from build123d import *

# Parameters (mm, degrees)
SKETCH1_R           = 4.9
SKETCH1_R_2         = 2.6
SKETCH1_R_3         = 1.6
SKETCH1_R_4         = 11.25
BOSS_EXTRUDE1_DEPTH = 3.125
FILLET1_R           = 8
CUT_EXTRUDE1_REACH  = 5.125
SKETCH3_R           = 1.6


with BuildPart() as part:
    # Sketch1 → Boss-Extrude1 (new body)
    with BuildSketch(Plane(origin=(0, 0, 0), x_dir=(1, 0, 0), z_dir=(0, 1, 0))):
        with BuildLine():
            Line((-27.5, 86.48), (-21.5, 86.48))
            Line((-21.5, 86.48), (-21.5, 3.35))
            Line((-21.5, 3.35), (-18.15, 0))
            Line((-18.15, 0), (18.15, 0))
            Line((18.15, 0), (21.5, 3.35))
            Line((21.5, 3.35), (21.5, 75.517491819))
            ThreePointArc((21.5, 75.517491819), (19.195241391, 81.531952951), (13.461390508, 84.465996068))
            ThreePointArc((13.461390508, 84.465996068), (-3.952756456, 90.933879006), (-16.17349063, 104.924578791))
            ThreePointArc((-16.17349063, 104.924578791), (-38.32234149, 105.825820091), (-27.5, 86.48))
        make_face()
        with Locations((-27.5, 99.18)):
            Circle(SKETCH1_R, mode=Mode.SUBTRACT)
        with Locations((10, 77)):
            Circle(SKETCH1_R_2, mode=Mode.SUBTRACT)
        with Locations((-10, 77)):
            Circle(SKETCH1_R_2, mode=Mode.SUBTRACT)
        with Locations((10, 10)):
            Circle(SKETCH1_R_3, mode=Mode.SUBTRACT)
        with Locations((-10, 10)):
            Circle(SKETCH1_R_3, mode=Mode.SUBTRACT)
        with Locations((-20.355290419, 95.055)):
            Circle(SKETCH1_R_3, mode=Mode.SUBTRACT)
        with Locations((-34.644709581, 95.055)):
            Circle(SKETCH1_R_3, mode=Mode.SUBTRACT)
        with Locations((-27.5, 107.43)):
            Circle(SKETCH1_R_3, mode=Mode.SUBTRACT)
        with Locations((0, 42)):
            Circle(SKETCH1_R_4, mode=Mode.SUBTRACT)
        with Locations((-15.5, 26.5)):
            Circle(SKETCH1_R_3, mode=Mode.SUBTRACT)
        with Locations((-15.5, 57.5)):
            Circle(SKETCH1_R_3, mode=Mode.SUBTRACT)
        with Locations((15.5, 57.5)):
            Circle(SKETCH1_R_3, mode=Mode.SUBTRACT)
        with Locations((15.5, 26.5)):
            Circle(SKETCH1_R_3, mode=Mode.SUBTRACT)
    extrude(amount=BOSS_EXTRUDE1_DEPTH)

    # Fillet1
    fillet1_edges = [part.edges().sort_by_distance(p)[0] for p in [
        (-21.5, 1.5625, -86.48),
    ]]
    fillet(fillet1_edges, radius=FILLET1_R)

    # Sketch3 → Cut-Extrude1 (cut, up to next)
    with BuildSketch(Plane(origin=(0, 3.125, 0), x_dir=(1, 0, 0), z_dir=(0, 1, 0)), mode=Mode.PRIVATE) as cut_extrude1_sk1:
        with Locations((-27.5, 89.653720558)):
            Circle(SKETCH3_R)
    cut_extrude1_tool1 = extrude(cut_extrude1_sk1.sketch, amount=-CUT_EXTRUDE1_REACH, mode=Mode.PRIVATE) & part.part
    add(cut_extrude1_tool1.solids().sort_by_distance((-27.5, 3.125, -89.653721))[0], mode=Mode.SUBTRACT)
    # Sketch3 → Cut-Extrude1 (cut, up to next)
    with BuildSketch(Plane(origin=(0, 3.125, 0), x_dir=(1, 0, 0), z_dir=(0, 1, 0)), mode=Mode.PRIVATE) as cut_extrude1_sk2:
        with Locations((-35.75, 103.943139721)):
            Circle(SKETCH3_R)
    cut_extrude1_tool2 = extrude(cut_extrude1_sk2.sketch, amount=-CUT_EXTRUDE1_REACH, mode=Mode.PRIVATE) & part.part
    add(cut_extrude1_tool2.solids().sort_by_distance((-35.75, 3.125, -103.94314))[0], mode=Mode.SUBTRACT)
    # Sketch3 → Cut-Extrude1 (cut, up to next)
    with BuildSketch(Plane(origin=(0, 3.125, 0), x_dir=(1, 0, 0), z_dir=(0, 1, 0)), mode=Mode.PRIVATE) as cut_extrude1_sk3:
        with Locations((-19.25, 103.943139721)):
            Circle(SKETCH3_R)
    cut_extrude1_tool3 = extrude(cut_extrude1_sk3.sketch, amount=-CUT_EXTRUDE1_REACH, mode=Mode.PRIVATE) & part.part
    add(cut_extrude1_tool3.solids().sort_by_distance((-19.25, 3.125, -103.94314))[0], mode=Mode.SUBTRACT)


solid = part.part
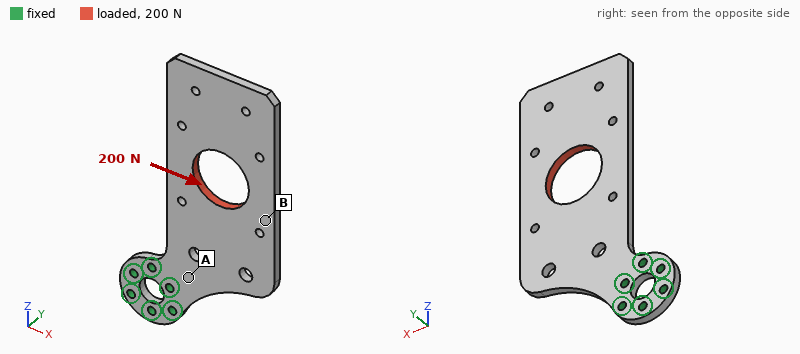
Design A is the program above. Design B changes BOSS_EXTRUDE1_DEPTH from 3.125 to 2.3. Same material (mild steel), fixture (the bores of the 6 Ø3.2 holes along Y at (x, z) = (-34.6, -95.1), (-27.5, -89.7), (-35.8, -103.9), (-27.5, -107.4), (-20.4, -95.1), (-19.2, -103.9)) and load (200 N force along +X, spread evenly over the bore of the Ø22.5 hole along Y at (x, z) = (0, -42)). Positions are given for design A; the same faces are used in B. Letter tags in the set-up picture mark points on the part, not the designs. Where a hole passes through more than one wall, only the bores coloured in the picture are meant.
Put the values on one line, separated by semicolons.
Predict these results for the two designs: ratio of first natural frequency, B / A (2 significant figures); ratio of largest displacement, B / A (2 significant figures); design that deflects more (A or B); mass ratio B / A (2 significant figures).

0.74; 1.4; B; 0.74
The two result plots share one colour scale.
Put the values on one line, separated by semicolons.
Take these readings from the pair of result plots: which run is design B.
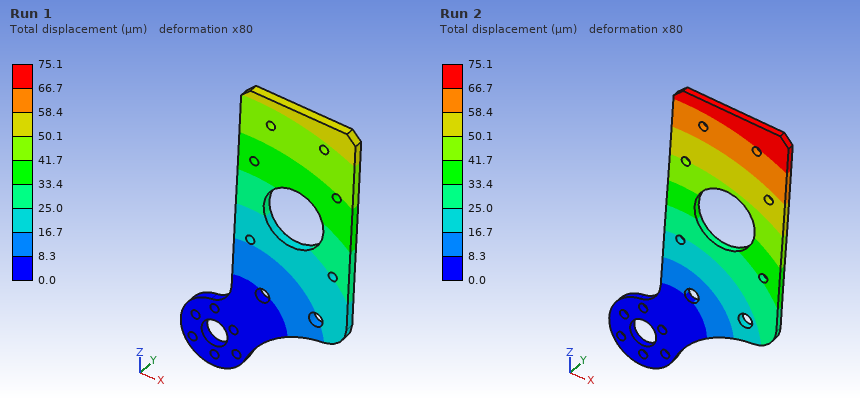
Run 2
